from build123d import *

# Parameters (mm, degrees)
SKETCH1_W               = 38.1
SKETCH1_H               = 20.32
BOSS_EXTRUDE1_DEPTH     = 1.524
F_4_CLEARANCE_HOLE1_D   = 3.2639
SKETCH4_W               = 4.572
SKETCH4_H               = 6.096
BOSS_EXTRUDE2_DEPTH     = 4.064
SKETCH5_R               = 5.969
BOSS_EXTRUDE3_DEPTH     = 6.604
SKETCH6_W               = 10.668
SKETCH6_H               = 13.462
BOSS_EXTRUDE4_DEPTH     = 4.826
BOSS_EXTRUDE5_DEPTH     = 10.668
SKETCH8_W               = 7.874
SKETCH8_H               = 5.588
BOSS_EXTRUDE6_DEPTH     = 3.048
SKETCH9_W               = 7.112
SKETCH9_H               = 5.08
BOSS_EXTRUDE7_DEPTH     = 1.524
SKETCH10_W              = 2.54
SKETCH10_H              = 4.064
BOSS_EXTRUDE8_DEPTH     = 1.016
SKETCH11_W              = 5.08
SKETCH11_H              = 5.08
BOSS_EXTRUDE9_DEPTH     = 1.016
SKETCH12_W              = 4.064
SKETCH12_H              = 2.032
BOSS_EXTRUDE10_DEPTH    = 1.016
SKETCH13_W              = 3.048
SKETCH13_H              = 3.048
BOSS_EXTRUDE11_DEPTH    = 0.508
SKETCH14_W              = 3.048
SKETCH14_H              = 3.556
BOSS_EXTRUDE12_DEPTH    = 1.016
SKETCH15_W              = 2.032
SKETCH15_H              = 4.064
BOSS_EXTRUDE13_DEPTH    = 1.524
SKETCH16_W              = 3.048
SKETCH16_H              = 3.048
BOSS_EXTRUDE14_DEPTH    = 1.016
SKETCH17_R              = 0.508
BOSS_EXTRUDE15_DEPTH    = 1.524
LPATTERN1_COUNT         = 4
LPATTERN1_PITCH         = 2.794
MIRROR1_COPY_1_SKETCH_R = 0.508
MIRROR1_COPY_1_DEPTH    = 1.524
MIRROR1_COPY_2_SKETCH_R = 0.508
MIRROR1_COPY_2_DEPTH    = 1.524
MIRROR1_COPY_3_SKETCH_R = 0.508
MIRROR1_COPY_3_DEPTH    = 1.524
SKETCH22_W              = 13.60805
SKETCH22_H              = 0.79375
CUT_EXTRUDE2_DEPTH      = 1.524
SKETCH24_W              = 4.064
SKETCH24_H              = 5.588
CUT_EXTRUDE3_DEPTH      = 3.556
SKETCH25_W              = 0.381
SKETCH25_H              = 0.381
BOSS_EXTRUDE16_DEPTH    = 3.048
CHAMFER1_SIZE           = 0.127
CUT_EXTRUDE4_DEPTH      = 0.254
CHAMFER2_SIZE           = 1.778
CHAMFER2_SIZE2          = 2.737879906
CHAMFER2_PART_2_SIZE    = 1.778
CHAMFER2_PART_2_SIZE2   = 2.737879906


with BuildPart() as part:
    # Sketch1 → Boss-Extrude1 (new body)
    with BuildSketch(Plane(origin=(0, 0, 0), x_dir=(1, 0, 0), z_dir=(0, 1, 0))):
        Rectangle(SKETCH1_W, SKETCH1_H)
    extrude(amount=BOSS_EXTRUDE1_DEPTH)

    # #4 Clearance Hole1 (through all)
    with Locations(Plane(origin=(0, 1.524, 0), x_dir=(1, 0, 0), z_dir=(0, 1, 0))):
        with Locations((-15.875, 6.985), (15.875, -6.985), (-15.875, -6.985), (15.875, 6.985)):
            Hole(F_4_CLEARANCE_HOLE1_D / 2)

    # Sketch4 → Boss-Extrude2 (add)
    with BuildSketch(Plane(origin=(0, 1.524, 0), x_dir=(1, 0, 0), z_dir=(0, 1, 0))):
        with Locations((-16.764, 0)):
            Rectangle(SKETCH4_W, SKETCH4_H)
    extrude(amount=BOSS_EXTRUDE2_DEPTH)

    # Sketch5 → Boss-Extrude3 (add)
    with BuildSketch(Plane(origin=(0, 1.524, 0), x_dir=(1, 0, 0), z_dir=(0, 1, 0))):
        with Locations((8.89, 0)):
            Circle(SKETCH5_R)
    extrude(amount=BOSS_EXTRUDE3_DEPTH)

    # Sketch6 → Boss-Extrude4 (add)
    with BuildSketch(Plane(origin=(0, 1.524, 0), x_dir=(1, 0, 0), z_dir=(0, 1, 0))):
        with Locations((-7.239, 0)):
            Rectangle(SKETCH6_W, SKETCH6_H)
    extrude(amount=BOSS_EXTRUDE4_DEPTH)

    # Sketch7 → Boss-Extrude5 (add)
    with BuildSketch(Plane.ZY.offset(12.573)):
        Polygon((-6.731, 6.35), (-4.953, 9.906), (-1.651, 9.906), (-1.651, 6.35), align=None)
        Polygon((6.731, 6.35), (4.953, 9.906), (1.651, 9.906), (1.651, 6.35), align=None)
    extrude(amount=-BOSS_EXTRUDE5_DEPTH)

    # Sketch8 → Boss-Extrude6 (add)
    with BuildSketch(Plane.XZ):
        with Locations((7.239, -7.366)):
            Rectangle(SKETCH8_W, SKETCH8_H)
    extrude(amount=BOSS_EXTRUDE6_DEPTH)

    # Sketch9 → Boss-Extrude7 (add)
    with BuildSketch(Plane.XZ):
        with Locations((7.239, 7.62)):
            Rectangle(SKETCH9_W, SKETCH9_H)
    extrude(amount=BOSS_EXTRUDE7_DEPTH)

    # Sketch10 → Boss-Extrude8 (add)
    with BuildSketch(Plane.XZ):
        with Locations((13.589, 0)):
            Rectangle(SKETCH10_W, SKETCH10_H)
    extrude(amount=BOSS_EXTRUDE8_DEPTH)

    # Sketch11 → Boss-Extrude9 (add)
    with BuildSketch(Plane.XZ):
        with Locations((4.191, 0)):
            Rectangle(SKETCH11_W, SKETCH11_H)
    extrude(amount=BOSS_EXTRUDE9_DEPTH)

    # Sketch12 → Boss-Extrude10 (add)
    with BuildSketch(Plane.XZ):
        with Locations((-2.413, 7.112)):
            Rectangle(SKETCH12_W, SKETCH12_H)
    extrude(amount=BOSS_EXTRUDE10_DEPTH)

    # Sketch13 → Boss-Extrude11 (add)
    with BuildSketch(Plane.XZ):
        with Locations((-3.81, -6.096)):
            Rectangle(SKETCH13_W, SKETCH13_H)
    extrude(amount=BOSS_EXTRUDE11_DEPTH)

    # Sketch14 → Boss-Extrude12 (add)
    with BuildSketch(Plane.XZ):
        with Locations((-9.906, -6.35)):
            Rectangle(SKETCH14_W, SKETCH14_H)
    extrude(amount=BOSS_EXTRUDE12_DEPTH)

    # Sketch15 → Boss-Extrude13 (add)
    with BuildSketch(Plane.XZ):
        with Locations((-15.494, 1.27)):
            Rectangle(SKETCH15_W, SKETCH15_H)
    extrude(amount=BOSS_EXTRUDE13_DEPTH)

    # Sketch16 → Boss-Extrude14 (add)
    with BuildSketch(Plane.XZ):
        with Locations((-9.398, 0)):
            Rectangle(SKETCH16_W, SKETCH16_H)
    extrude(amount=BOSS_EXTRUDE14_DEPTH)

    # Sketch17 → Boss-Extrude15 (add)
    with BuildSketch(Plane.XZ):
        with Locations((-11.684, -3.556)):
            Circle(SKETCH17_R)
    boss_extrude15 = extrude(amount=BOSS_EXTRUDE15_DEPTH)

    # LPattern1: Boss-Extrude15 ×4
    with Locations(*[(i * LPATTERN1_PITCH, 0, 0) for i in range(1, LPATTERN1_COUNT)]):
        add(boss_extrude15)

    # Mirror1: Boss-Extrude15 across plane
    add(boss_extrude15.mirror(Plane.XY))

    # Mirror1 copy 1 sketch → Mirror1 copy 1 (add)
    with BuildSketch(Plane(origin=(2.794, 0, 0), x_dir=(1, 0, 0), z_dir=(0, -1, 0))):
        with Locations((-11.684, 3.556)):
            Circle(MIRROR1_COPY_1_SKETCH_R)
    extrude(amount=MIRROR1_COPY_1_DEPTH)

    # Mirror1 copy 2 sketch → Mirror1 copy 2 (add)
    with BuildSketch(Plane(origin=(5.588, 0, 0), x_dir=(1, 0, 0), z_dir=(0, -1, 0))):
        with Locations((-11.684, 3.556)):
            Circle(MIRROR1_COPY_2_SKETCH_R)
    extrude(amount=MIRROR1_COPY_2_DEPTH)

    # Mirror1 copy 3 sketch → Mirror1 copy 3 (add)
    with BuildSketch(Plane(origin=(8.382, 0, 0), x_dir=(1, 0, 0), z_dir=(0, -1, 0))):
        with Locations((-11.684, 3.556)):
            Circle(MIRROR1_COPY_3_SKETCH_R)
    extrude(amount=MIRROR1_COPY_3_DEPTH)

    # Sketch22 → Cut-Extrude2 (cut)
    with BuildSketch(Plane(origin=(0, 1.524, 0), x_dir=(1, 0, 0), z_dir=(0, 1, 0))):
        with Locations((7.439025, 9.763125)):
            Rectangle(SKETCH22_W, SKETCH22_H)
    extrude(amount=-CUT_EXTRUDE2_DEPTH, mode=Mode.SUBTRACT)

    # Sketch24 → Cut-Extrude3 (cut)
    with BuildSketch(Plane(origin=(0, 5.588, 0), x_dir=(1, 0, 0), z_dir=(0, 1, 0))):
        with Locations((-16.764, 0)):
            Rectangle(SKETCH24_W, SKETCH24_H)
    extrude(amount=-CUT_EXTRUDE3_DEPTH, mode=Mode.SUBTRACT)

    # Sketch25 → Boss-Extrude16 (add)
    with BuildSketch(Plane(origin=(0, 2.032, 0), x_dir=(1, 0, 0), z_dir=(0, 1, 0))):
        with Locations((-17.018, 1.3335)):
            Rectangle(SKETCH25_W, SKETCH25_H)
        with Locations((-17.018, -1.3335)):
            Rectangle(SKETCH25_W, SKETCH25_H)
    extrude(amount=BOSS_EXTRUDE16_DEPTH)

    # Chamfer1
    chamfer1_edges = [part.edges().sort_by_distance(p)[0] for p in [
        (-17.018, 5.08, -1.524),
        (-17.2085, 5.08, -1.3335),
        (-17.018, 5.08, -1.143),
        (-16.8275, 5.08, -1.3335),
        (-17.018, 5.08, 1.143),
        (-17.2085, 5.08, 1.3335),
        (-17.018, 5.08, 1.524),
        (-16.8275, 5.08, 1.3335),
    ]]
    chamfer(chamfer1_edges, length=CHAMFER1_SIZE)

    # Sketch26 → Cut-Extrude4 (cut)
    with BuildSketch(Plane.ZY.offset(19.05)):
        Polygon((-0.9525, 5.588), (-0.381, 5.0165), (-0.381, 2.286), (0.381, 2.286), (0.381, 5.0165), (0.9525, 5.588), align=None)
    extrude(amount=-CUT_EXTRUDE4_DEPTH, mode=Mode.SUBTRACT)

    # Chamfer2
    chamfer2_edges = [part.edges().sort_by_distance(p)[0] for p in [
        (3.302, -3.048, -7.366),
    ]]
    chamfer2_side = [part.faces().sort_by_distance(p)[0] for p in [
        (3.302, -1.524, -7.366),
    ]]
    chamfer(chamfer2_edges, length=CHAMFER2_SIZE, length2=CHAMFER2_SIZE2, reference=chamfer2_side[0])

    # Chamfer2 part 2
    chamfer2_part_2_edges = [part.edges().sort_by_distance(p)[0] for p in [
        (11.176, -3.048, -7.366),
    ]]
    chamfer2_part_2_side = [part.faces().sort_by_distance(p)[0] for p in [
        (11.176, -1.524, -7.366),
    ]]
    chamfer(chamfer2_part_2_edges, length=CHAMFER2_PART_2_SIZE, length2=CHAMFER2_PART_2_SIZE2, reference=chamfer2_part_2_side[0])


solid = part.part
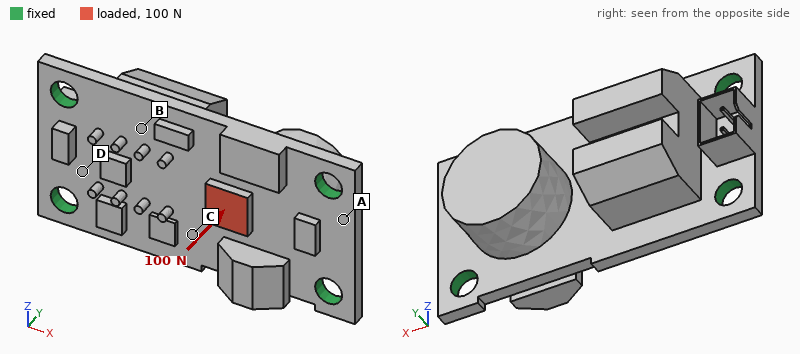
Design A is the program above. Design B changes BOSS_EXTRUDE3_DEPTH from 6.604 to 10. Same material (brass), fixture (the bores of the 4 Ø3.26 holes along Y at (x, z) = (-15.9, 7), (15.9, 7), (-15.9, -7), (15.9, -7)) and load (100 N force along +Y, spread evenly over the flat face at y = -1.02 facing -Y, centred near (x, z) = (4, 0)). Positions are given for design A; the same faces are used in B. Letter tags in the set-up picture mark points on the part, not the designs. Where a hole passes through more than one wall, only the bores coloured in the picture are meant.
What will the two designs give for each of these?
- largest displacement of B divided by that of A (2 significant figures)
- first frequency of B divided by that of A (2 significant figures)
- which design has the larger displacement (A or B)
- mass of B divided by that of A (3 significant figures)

1.1
0.90
B
1.12
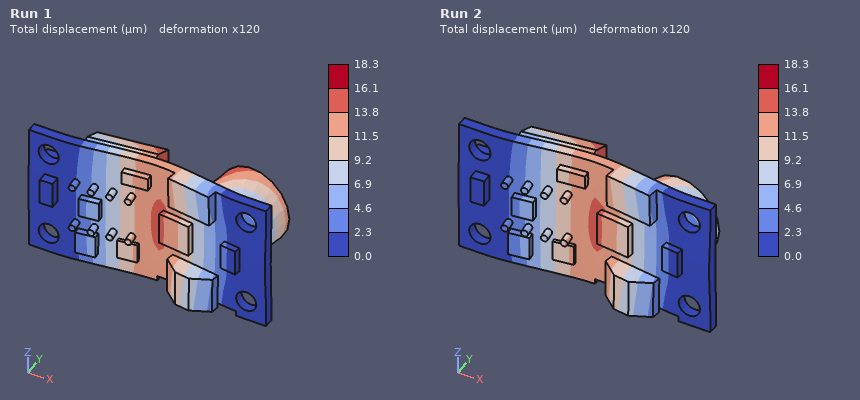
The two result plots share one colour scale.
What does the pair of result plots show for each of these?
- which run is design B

Run 1
